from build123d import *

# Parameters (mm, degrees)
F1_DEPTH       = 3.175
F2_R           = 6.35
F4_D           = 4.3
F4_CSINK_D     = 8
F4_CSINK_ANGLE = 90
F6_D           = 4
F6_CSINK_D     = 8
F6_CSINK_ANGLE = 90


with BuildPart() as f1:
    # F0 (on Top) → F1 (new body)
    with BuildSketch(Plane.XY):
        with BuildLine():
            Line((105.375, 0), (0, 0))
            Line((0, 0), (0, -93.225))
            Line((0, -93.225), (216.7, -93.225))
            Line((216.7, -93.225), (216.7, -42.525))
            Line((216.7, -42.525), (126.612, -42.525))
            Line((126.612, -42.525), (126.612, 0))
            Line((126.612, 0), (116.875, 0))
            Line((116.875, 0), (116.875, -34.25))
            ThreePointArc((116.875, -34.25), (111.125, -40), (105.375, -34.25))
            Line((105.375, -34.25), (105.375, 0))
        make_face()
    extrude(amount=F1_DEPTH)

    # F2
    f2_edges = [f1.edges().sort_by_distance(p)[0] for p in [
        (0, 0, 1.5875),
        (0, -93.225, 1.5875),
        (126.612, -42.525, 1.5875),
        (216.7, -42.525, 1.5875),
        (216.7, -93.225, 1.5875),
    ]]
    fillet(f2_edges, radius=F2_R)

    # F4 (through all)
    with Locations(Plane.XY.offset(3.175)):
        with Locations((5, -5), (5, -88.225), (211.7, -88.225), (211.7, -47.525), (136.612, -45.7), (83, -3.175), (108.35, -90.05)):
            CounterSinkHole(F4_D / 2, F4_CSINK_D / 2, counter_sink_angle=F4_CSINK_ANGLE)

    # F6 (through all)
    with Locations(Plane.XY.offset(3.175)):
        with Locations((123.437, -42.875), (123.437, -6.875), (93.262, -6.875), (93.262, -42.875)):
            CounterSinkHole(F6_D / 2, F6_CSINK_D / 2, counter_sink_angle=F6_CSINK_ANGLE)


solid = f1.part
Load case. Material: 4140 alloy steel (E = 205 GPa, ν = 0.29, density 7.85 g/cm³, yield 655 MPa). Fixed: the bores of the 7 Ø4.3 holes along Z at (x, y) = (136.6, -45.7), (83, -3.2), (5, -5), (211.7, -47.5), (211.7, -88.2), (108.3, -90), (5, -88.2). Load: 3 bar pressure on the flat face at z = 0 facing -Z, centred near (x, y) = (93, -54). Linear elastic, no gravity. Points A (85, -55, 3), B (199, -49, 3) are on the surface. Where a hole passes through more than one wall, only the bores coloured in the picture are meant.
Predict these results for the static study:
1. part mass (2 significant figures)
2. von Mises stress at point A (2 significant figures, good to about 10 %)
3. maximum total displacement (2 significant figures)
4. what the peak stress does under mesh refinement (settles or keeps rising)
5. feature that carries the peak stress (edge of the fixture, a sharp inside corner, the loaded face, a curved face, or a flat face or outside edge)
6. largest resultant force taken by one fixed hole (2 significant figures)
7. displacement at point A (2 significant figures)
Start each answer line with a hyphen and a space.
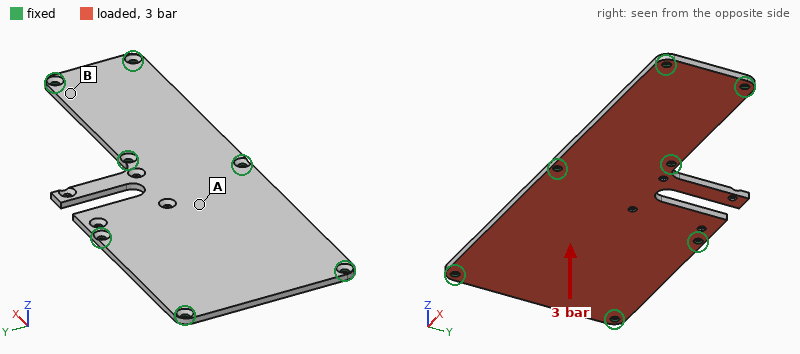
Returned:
- 390 g
- 77 MPa
- 0.38 mm
- keeps rising
- edge of the fixture
- 1.8 kN
- 0.22 mm
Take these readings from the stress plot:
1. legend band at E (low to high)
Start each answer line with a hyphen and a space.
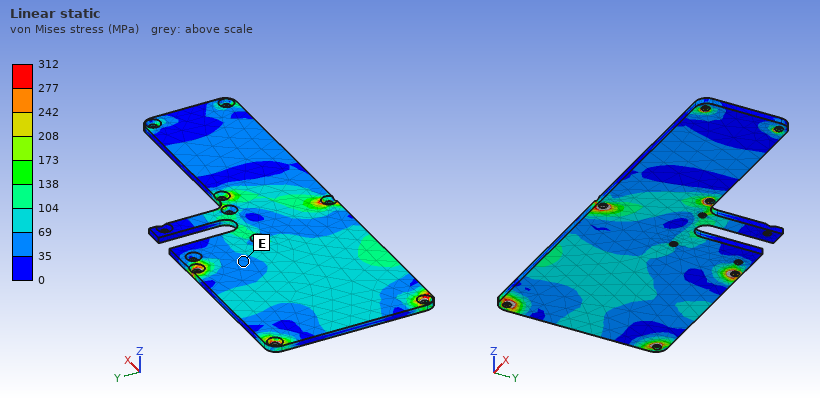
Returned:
- 35 to 69 MPa
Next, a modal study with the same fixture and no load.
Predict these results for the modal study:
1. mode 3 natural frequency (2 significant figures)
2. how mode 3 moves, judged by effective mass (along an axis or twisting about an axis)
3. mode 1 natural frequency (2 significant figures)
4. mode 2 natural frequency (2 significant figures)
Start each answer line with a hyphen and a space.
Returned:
- 1700 Hz
- along Z
- 1100 Hz
- 1200 Hz
